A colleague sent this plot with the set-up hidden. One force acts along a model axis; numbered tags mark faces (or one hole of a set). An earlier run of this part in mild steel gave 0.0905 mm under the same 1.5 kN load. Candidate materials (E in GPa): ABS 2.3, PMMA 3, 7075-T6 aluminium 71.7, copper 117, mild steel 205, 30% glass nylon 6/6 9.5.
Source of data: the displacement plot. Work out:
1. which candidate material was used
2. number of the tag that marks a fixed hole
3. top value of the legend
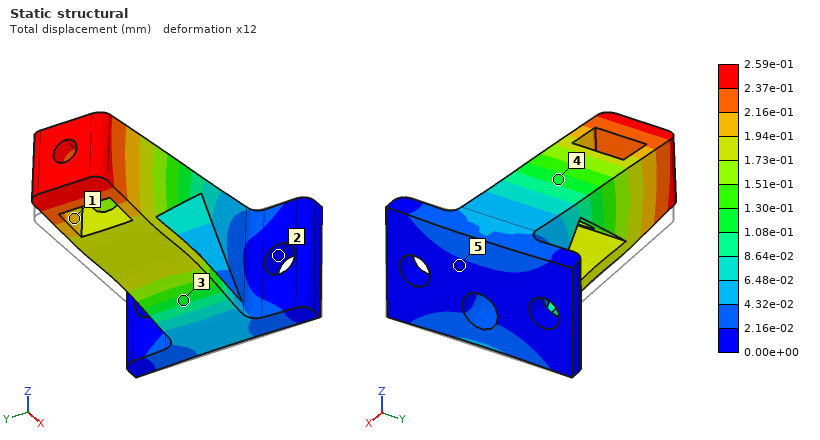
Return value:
7075-T6 aluminium
2
2.59e-01 mm
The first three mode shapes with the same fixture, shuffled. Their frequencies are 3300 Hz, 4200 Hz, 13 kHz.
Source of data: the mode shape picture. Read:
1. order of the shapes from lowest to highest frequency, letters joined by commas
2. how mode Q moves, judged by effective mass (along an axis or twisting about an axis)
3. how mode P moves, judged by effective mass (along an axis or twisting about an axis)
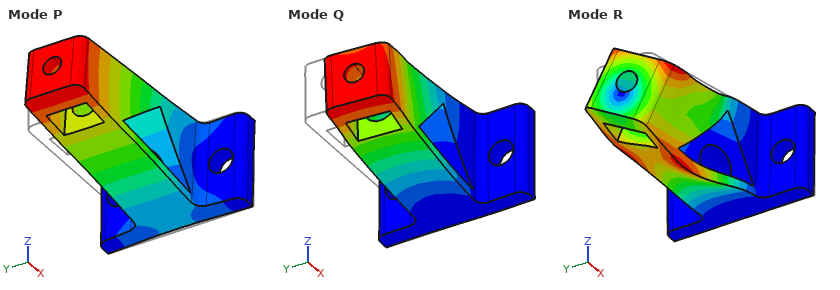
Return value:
P, Q, R
along Y
along Z
